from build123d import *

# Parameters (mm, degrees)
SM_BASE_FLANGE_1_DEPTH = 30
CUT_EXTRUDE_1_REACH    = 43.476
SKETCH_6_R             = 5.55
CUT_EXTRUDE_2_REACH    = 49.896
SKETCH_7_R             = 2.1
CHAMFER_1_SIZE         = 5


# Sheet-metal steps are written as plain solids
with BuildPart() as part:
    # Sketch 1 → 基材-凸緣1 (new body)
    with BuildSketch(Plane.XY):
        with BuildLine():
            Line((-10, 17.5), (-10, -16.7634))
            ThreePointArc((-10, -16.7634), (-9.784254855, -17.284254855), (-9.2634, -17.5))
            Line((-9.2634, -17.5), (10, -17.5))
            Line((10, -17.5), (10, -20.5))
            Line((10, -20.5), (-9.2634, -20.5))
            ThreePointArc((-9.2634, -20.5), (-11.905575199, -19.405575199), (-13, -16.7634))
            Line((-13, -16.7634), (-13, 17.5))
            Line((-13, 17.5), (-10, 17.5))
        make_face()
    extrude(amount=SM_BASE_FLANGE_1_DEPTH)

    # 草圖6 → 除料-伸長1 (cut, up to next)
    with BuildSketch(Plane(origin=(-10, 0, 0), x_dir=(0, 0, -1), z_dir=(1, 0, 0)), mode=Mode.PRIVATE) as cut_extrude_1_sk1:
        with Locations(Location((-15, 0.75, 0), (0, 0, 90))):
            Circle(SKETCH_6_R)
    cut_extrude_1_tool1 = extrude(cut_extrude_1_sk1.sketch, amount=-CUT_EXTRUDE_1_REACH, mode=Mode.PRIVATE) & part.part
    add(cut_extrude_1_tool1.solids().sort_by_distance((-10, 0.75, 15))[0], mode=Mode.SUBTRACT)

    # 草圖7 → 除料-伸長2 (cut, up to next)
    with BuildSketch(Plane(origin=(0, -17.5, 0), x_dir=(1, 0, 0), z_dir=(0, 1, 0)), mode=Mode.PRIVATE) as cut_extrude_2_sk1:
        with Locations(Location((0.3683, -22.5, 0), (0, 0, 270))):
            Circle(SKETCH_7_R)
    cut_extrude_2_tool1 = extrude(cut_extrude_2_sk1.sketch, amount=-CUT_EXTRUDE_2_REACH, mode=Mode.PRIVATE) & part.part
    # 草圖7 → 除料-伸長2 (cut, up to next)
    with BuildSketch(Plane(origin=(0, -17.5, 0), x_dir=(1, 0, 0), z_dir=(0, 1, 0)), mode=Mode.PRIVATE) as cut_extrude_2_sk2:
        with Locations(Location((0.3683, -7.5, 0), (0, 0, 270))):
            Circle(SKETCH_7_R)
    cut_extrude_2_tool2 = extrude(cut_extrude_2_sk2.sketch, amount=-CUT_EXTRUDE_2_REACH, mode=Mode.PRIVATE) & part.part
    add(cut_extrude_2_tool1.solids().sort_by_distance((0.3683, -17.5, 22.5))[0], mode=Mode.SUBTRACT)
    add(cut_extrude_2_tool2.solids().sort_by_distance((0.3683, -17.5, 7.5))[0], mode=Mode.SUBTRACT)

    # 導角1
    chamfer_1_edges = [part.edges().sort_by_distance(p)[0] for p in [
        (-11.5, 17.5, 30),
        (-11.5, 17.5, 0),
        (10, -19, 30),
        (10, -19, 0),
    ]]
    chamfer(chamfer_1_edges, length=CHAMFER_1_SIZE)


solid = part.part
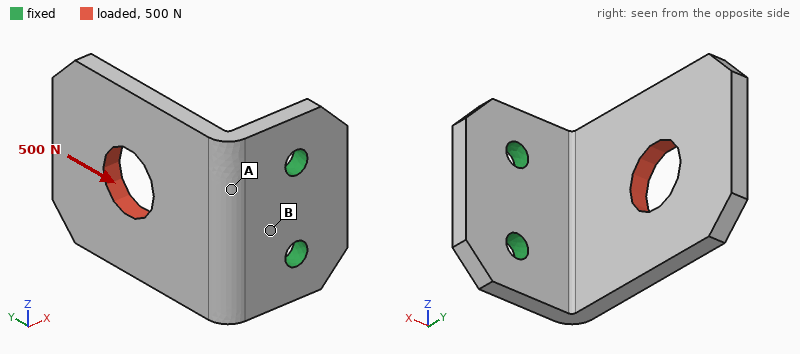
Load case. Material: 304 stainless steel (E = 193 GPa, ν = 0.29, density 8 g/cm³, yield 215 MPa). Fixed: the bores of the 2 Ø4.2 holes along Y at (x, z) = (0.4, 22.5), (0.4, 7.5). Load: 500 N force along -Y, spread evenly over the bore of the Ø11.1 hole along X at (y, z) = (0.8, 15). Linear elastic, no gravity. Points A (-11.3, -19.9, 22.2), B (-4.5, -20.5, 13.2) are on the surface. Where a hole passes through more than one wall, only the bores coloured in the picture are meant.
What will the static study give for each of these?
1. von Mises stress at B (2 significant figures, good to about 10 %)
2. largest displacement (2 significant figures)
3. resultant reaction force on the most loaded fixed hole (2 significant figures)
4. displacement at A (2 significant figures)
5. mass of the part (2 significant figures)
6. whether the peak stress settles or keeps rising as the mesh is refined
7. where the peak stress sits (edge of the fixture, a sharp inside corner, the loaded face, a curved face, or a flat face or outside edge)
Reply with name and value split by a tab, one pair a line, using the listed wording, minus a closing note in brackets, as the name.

von Mises stress at B	62 MPa
largest displacement	87 µm
resultant reaction force on the most loaded fixed hole	250 N
displacement at A	18 µm
mass of the part	37 g
whether the peak stress settles or keeps rising as the mesh is refined	keeps rising
where the peak stress sits	edge of the fixture
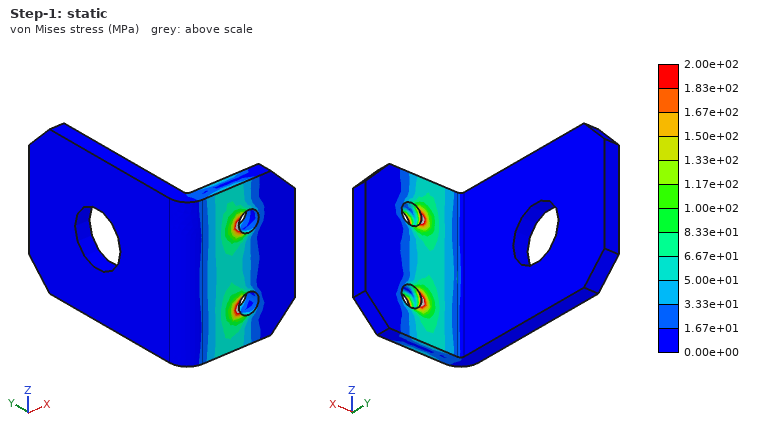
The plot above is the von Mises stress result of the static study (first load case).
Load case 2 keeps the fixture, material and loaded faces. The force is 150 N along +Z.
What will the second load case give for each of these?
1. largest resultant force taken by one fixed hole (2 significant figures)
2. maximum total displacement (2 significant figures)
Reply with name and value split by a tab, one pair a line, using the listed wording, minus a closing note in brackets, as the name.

largest resultant force taken by one fixed hole	190 N
maximum total displacement	25 µm
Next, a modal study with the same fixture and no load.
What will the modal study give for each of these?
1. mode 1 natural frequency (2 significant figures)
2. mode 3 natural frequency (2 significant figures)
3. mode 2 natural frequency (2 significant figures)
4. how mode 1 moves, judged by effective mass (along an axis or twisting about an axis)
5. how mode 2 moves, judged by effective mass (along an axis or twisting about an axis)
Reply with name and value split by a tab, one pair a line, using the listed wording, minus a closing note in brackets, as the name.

mode 1 natural frequency	1300 Hz
mode 3 natural frequency	4900 Hz
mode 2 natural frequency	3100 Hz
how mode 1 moves, judged by effective mass	along X
how mode 2 moves, judged by effective mass	along Z
